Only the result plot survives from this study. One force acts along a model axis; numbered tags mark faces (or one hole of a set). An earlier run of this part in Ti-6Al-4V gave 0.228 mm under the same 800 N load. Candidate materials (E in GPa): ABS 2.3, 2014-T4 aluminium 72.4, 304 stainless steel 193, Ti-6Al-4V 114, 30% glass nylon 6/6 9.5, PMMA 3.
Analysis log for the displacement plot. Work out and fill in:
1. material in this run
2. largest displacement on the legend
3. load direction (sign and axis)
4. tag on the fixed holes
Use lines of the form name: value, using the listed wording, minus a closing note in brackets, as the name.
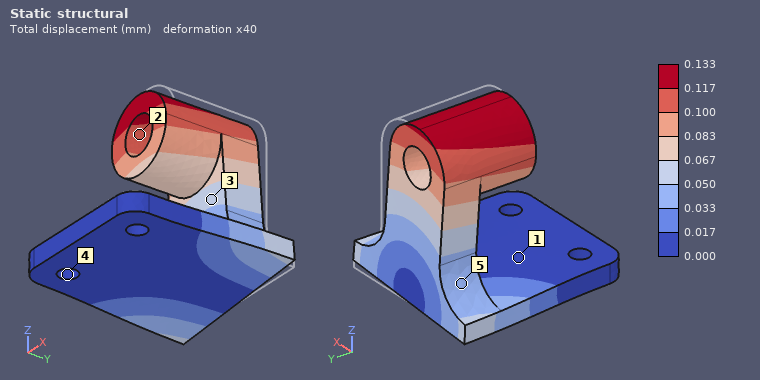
material in this run: 304 stainless steel
largest displacement on the legend: 0.133 mm
load direction: -X
tag on the fixed holes: 4
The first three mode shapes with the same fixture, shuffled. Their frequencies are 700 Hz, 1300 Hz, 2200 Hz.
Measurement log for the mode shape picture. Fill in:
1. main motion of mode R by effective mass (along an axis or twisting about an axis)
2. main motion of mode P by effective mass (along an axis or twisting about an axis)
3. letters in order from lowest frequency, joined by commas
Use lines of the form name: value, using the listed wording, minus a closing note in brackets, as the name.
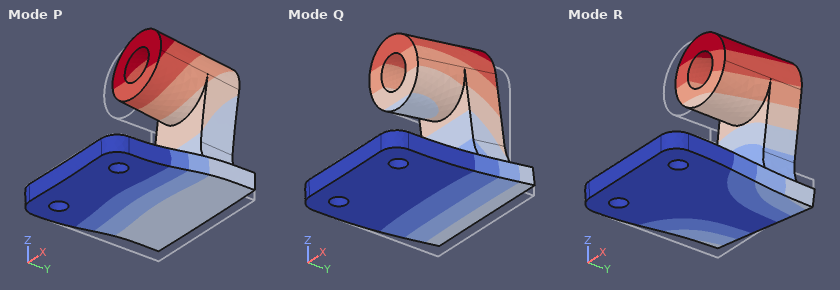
main motion of mode R by effective mass: along X
main motion of mode P by effective mass: along Z
letters in order from lowest frequency, joined by commas: Q, R, P
